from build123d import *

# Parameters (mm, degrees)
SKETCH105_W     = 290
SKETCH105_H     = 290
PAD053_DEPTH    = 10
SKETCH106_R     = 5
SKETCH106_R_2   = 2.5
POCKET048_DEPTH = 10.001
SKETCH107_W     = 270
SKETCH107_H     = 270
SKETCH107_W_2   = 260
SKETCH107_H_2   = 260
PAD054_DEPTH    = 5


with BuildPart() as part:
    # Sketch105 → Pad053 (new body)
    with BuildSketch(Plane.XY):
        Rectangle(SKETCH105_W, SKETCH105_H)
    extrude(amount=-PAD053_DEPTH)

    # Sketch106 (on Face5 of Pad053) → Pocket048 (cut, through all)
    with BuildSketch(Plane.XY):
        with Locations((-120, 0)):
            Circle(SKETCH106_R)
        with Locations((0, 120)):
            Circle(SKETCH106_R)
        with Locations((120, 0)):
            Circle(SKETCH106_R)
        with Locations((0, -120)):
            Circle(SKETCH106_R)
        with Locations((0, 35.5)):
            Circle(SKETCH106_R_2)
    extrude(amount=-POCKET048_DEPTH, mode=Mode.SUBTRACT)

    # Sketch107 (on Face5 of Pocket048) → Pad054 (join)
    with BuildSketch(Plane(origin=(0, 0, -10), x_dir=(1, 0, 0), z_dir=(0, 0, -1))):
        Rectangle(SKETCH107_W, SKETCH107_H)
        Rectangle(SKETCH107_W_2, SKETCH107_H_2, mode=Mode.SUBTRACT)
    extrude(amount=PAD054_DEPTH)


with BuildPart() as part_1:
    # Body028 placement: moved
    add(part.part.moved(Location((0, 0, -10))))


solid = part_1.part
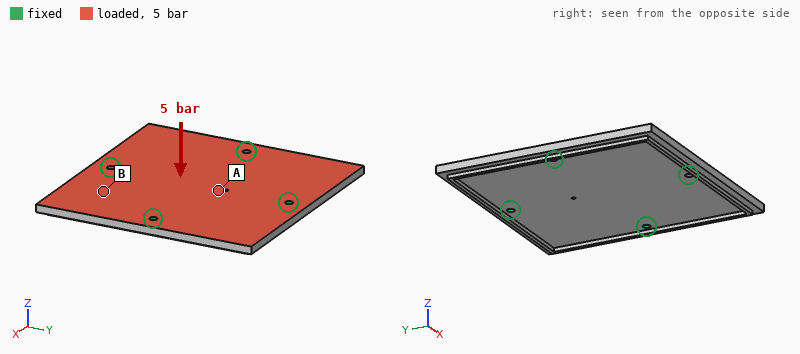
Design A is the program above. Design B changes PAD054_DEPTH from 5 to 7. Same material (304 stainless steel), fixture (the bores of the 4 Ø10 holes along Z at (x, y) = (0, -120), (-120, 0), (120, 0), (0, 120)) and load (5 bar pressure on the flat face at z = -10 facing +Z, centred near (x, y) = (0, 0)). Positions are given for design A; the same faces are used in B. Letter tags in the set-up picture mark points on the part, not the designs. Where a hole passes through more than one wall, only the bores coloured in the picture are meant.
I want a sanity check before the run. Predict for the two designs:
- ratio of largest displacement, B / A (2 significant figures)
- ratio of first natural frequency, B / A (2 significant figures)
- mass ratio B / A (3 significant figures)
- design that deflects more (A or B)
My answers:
0.89
1.0
1.01
A
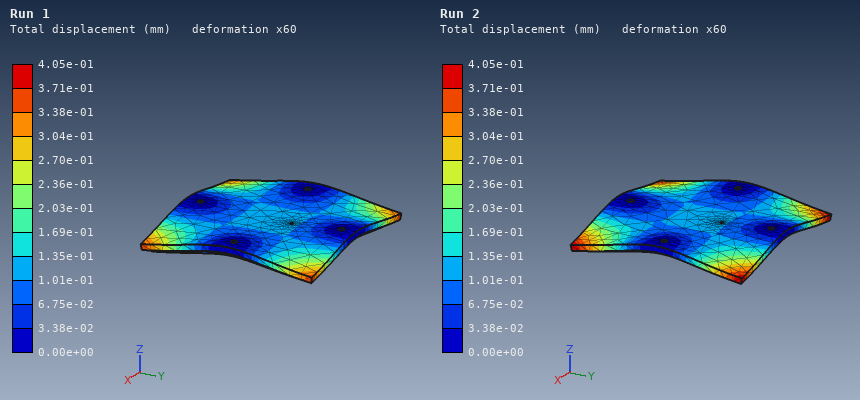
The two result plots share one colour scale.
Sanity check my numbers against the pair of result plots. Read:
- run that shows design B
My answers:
Run 1
